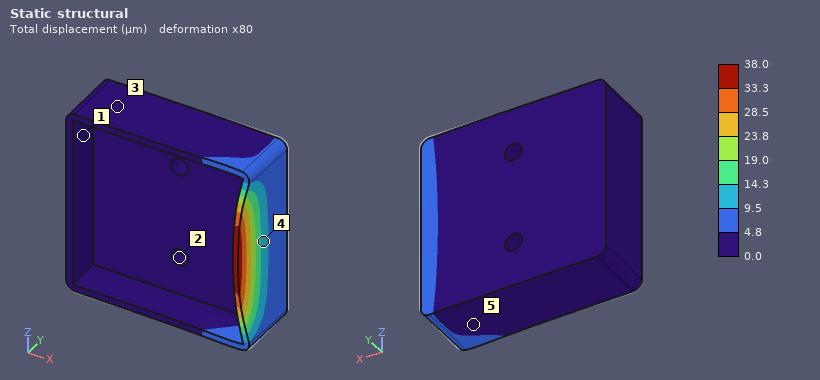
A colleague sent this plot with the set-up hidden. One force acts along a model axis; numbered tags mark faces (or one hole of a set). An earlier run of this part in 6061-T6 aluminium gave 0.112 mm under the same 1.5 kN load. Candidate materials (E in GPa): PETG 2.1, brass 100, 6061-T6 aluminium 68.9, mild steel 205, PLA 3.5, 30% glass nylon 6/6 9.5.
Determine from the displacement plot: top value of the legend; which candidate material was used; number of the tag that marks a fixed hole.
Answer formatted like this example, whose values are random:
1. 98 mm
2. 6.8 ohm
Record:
1. 38.0 µm
2. mild steel
3. 2
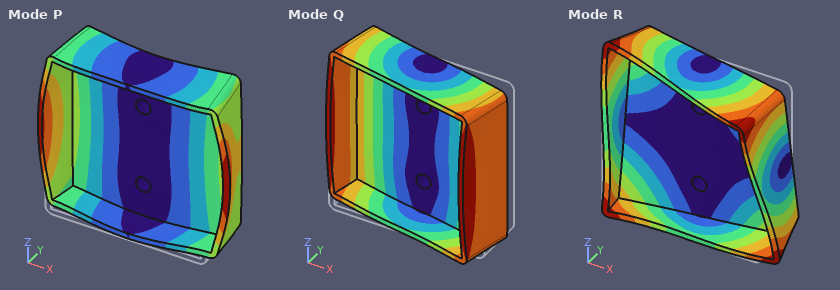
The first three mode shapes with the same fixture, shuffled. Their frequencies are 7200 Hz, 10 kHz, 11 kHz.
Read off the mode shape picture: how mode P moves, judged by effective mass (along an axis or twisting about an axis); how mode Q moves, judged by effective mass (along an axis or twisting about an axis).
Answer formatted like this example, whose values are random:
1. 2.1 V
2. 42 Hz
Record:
1. along Y
2. twisting about Z
